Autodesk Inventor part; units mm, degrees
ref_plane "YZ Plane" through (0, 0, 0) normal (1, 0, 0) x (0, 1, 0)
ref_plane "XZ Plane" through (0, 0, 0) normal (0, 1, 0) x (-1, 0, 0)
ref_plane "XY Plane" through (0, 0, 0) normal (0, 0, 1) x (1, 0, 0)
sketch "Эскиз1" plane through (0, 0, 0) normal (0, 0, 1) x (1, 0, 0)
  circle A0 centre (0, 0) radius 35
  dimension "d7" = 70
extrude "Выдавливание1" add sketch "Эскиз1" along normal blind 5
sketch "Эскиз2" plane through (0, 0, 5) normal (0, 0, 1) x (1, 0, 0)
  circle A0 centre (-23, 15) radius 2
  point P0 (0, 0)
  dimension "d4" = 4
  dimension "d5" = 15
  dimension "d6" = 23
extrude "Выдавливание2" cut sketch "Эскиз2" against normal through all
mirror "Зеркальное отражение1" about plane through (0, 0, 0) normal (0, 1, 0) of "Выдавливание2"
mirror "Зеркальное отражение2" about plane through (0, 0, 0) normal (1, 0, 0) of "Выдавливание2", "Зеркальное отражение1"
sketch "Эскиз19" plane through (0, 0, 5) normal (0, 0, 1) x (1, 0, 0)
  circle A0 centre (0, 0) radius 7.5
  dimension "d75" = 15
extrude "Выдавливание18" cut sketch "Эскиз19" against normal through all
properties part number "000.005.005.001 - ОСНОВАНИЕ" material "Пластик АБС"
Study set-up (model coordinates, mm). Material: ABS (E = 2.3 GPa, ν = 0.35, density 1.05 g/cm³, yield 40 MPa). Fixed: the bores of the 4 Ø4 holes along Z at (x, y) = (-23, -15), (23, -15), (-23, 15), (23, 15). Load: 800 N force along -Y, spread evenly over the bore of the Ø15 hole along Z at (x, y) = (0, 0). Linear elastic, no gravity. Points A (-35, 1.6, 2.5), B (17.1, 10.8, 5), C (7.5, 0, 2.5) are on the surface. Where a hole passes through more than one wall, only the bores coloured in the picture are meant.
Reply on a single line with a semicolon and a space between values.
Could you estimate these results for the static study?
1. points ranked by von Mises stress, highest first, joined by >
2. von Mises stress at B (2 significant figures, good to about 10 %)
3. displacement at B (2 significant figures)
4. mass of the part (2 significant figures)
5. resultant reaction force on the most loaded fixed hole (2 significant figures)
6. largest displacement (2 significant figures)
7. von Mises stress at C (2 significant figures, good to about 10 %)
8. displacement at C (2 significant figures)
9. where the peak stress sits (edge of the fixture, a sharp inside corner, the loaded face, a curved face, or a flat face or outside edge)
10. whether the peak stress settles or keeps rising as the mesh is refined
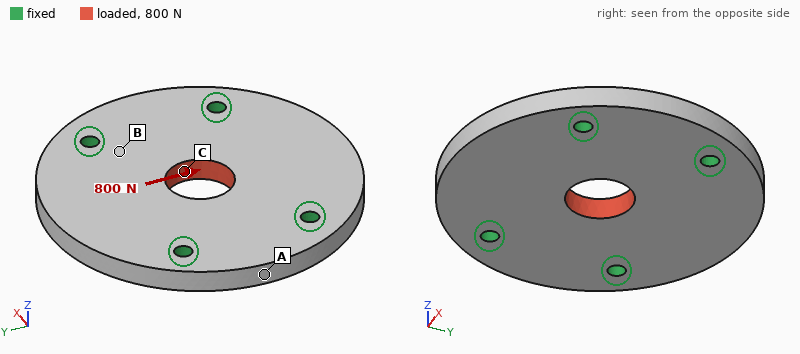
C > B > A; 3.2 MPa; 13 µm; 19 g; 210 N; 45 µm; 5.9 MPa; 38 µm; edge of the fixture; keeps rising
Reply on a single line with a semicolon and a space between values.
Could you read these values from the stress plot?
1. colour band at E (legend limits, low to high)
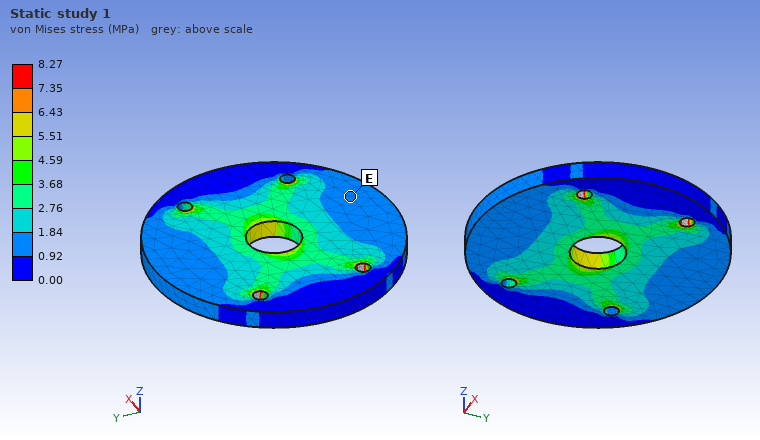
0.92 to 1.84 MPa
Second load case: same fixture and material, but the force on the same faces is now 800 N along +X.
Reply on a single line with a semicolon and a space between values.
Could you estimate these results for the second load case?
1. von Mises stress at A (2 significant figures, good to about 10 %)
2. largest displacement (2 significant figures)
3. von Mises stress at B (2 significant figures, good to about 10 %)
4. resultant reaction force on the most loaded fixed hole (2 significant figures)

1.4 MPa; 30 µm; 3.3 MPa; 210 N
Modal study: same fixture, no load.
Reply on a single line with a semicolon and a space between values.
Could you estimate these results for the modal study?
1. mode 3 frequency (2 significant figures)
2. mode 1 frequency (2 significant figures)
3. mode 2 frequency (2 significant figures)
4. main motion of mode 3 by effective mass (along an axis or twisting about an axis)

3600 Hz; 2300 Hz; 2300 Hz; along Z
